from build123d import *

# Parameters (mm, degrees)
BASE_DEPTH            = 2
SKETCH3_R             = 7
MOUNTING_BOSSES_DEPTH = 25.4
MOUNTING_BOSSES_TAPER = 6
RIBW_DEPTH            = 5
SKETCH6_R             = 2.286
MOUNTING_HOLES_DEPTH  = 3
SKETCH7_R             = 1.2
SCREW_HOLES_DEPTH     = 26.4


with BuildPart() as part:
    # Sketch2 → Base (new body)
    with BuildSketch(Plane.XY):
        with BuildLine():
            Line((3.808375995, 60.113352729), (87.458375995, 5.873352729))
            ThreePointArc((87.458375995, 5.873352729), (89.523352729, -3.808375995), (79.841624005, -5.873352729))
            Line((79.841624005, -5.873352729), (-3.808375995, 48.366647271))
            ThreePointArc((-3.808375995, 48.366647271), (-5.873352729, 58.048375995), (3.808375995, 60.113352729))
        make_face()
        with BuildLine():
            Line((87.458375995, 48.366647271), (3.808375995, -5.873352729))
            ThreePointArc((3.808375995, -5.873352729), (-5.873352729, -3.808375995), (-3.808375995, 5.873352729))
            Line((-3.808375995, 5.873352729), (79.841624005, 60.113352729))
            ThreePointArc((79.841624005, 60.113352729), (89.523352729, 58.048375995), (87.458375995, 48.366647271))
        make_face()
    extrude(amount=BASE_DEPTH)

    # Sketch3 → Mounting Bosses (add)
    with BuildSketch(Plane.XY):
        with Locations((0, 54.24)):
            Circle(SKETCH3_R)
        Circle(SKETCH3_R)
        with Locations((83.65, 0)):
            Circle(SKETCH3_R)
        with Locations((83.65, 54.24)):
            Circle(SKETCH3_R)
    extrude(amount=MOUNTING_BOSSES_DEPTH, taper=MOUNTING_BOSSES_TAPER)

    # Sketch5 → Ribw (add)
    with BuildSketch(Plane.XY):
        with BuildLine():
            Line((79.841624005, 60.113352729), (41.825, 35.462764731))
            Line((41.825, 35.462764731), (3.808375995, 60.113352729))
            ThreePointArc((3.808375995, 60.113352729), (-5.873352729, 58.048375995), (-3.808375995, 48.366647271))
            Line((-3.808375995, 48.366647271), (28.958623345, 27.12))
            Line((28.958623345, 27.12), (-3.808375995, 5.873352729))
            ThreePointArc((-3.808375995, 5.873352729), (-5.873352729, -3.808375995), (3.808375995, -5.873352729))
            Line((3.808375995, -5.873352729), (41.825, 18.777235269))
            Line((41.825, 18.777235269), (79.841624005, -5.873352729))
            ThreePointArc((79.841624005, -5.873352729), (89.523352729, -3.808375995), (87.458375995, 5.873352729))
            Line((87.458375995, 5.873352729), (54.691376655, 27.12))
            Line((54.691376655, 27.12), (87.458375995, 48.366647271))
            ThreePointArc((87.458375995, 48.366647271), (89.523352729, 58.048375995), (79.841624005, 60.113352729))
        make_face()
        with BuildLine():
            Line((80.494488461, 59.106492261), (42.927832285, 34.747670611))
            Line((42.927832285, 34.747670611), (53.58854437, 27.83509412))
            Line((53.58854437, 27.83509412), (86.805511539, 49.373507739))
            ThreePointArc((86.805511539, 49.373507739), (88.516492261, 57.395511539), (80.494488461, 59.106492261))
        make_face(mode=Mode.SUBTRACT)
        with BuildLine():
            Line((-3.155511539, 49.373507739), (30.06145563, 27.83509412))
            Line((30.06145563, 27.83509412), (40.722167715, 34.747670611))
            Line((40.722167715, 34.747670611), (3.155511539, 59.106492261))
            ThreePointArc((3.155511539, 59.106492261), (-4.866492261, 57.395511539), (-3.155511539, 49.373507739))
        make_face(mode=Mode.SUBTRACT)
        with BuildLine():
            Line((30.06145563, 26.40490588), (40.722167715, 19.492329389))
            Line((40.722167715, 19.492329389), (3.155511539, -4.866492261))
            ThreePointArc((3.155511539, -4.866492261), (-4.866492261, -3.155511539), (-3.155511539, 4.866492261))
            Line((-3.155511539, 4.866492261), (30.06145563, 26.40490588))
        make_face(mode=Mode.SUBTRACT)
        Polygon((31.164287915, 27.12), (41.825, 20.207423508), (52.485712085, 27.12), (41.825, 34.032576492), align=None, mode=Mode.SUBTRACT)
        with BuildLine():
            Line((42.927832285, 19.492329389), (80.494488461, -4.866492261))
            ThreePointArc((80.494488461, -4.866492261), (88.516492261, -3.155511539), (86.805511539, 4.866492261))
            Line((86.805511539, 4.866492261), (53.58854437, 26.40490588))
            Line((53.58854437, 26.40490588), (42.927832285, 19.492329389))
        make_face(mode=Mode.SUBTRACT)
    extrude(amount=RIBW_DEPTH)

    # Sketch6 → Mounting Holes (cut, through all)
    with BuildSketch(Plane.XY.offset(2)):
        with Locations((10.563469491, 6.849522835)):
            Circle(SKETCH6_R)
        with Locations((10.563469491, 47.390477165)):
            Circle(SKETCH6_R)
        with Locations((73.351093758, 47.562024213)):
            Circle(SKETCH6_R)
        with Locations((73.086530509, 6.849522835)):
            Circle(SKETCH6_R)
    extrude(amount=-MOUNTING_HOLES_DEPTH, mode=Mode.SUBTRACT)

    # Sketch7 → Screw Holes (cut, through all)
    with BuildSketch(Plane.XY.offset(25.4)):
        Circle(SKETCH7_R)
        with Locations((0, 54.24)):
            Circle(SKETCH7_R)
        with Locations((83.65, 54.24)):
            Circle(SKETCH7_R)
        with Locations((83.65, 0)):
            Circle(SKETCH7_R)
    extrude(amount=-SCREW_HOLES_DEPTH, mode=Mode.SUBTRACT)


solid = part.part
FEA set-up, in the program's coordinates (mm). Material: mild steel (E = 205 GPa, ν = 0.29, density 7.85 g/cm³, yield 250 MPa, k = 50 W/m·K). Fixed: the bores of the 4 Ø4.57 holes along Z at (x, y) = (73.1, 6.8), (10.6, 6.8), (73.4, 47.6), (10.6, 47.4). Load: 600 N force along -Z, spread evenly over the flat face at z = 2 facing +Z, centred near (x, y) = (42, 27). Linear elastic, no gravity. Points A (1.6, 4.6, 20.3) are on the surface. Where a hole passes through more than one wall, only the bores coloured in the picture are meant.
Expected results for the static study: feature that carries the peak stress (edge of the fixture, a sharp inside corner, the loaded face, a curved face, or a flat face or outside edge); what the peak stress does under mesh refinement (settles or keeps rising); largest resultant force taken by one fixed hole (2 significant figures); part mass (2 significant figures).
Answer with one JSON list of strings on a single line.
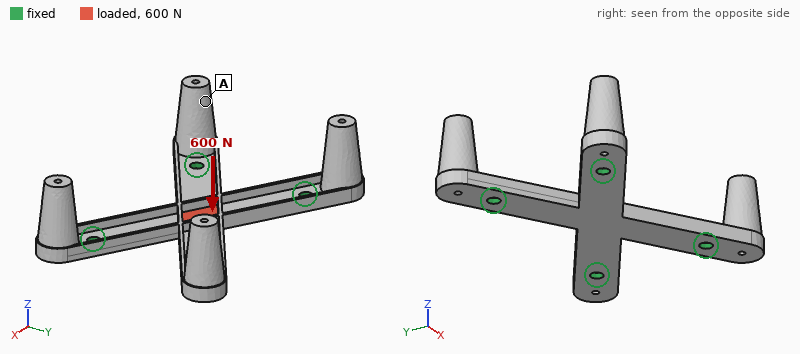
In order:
["edge of the fixture", "keeps rising", "200 N", "120 g"]
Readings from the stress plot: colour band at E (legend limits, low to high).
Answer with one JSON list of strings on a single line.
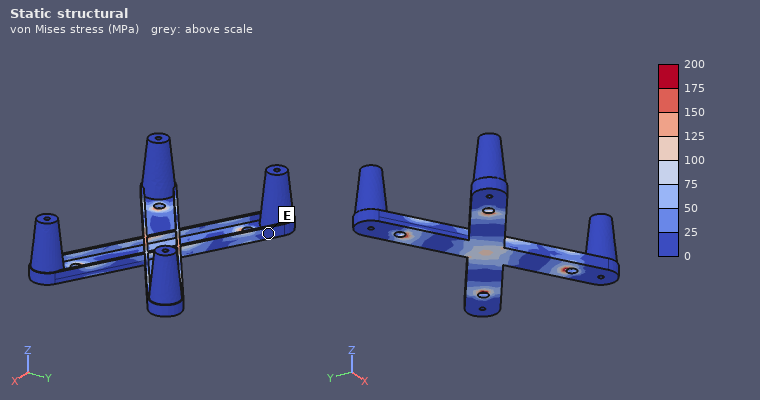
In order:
["0 to 25 MPa"]
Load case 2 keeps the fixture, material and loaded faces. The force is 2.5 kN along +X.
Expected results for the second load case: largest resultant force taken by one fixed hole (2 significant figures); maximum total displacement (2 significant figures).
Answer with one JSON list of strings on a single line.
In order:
["730 N", "5.5 µm"]
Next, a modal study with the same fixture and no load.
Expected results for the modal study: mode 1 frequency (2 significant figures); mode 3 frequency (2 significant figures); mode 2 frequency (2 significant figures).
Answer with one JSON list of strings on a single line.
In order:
["2100 Hz", "2200 Hz", "2200 Hz"]
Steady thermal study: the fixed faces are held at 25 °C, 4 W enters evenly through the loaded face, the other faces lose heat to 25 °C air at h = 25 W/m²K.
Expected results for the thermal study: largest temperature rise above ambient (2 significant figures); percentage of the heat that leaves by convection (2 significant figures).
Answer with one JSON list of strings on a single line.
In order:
["18 K", "28 %"]
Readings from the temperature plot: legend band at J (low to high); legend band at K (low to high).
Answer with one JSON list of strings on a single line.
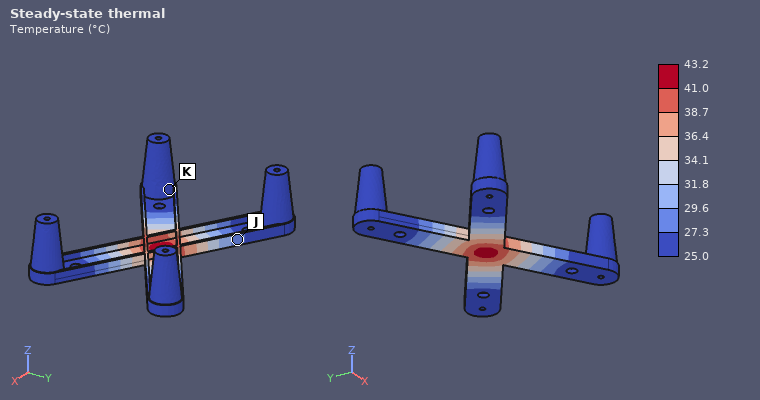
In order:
["27.3 to 29.6 °C", "25.0 to 27.3 °C"]
